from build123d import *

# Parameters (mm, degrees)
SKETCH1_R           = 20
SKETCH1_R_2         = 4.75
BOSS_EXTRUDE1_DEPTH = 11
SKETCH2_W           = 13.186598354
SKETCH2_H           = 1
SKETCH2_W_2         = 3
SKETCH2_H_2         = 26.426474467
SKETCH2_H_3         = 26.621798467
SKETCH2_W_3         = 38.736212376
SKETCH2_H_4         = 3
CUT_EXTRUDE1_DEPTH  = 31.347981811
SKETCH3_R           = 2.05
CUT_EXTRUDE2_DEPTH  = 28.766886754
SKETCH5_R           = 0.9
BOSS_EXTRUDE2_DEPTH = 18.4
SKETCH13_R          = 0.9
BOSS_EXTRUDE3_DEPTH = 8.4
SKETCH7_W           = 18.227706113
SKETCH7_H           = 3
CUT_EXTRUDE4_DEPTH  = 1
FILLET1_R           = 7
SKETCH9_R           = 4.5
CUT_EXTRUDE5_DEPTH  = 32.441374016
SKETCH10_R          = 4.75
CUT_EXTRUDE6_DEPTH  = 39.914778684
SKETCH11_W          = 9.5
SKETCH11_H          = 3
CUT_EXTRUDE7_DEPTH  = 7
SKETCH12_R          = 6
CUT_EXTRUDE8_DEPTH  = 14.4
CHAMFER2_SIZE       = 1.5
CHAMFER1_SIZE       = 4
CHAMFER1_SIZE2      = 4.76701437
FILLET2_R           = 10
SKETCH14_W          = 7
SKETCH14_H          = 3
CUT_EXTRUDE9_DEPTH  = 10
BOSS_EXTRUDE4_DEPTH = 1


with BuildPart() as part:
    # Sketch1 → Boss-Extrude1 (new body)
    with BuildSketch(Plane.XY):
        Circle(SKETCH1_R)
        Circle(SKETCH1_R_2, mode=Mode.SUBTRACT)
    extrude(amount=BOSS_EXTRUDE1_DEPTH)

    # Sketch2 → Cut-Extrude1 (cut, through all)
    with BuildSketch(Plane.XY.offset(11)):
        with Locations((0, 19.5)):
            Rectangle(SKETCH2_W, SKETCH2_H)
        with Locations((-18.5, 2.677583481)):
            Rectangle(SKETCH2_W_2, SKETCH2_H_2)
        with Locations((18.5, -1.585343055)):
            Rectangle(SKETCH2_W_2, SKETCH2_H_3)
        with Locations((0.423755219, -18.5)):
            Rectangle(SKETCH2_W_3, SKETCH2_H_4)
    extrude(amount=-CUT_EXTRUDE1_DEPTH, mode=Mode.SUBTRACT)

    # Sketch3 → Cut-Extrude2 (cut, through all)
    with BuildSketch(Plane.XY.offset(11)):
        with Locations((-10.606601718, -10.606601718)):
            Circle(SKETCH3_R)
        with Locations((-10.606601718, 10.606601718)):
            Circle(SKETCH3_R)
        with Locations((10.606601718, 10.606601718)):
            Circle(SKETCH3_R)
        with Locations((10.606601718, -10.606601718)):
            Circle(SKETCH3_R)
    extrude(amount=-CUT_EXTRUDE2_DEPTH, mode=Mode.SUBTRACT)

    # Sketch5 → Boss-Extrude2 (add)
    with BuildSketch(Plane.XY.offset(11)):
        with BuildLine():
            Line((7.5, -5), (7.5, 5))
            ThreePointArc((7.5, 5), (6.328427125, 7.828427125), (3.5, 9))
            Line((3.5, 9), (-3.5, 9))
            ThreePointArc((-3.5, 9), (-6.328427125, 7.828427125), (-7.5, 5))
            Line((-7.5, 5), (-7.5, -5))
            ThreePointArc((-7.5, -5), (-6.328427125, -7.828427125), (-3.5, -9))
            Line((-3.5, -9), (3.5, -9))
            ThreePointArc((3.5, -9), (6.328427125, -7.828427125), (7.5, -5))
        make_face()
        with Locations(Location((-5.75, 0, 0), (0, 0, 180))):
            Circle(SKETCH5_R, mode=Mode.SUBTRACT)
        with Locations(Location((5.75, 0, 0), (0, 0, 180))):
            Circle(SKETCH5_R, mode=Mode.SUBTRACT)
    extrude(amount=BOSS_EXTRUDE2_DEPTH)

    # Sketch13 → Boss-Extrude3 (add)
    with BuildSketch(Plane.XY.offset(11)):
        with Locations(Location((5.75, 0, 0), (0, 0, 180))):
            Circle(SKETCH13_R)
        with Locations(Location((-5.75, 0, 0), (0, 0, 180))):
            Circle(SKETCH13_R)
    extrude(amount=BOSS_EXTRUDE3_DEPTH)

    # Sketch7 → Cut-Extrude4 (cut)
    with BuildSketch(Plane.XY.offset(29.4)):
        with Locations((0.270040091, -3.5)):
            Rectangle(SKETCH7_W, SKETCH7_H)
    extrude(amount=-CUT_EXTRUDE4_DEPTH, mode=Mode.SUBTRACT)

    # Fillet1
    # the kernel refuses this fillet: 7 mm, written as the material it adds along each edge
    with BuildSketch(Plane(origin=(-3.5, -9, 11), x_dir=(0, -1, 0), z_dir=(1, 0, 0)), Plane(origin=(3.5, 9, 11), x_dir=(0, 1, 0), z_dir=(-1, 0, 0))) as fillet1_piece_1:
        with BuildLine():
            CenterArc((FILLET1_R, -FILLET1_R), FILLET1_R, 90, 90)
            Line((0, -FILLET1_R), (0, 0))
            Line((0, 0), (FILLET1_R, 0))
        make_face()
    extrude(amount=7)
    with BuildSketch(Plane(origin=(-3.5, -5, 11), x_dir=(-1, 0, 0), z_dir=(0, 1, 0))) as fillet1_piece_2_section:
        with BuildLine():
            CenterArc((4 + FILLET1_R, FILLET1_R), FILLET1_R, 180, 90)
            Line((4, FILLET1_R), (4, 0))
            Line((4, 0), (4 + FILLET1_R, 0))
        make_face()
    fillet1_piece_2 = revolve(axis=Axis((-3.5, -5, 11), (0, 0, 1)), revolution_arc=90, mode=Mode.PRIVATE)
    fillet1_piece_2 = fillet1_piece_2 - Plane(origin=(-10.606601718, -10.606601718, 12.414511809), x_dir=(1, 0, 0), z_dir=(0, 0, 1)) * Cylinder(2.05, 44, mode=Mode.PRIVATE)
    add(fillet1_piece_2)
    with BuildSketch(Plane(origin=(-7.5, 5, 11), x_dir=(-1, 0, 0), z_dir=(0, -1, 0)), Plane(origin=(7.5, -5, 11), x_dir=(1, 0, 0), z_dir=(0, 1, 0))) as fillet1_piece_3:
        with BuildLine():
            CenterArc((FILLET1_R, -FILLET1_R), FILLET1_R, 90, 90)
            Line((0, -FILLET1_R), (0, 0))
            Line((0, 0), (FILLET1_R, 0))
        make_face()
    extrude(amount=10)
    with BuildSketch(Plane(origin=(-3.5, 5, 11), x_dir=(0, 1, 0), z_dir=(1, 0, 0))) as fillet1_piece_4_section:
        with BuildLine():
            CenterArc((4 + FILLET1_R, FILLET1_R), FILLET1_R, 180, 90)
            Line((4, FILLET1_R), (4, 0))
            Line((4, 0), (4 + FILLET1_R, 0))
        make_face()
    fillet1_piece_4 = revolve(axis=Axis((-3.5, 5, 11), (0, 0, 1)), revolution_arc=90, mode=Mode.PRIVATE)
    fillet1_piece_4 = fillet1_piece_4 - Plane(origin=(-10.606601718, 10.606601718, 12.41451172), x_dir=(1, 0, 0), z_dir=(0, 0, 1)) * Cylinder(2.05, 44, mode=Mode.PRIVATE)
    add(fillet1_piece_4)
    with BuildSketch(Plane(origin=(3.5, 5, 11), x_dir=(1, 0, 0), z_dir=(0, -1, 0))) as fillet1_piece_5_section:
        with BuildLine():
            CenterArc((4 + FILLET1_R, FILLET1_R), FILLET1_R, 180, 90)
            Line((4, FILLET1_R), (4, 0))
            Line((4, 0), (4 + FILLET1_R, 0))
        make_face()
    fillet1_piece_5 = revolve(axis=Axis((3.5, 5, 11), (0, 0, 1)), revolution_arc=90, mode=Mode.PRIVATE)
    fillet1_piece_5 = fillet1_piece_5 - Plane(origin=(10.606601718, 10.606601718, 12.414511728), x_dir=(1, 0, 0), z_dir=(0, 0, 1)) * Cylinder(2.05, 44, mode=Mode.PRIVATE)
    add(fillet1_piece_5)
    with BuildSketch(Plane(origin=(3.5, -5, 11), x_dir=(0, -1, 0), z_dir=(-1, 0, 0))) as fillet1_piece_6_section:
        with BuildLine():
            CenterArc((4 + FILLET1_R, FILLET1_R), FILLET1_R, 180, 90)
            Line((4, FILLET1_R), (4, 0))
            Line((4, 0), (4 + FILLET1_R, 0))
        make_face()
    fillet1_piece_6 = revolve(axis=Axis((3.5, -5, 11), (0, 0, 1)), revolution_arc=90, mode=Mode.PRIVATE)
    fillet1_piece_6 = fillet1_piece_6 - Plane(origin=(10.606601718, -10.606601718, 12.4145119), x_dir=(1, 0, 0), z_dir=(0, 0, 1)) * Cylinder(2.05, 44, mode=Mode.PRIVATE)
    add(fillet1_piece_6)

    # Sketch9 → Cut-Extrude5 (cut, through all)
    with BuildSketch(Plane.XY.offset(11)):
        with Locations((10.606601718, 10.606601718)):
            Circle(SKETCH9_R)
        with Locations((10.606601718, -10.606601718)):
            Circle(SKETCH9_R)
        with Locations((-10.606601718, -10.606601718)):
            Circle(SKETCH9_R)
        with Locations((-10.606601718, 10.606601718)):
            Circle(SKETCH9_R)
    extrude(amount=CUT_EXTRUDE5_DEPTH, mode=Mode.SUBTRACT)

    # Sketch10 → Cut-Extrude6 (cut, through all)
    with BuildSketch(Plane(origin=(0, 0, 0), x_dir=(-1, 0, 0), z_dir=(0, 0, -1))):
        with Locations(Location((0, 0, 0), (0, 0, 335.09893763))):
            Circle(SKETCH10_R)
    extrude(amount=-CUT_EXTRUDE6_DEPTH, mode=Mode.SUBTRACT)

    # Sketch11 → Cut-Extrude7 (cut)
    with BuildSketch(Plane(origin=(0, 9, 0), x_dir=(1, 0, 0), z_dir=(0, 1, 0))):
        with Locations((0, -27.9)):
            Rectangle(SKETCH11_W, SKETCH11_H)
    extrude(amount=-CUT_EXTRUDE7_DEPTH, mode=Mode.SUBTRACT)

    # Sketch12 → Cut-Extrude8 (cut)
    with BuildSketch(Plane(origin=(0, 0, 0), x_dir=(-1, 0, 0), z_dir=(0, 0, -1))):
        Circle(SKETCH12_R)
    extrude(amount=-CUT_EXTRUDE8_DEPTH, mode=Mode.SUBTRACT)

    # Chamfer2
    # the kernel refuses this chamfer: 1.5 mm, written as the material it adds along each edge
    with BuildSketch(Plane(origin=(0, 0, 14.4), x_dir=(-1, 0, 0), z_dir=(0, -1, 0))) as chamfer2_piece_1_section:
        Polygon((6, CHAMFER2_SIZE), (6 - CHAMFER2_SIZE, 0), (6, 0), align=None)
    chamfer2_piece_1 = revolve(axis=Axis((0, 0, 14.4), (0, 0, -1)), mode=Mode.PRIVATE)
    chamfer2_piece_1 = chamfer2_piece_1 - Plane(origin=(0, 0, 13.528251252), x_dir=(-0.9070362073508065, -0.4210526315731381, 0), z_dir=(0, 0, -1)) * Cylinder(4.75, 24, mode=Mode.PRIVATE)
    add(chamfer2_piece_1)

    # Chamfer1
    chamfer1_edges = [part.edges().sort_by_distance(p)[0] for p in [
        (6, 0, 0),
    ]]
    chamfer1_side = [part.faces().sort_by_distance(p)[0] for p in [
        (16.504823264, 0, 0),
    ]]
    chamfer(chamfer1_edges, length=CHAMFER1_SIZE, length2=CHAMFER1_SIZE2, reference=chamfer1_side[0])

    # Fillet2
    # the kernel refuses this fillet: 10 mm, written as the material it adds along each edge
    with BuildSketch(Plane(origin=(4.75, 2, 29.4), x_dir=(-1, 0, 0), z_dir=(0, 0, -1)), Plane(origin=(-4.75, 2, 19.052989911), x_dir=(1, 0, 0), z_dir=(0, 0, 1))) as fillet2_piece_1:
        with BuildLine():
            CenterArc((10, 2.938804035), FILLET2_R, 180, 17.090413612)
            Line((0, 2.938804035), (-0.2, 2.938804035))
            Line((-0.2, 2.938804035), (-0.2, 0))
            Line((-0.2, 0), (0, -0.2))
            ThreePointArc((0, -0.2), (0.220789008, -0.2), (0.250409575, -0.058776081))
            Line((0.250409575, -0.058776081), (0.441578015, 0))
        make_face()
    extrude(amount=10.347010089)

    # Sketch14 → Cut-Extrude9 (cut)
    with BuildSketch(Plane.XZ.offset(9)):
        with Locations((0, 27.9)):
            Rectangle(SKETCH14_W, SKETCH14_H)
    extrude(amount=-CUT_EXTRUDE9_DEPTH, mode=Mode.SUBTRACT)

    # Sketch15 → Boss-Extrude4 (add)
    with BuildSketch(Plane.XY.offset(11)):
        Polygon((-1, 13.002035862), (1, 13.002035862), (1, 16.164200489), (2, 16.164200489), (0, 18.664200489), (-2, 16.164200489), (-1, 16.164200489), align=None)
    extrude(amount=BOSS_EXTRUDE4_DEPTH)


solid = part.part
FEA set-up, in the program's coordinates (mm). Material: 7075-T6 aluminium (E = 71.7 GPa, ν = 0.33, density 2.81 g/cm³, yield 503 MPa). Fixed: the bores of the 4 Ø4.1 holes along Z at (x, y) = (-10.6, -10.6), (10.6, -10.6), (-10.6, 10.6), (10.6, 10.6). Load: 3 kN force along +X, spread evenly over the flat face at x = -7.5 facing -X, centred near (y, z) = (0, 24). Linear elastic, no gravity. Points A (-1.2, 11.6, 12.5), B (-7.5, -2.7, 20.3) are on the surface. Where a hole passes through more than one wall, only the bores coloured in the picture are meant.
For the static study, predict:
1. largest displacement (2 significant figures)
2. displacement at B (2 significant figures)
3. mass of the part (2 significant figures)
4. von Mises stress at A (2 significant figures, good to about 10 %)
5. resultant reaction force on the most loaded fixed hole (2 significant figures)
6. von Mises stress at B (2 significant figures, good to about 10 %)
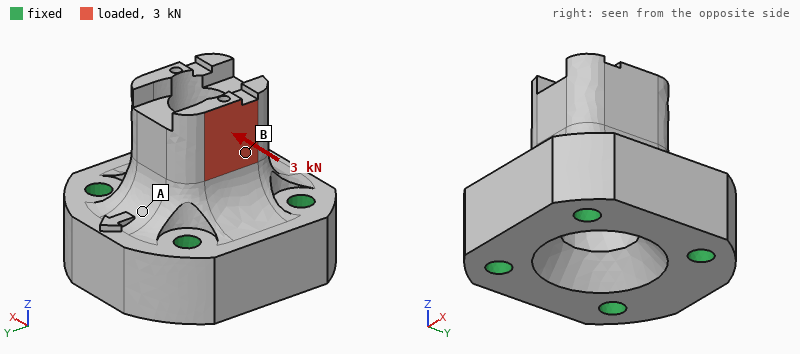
57 µm
21 µm
38 g
18 MPa
1.4 kN
54 MPa
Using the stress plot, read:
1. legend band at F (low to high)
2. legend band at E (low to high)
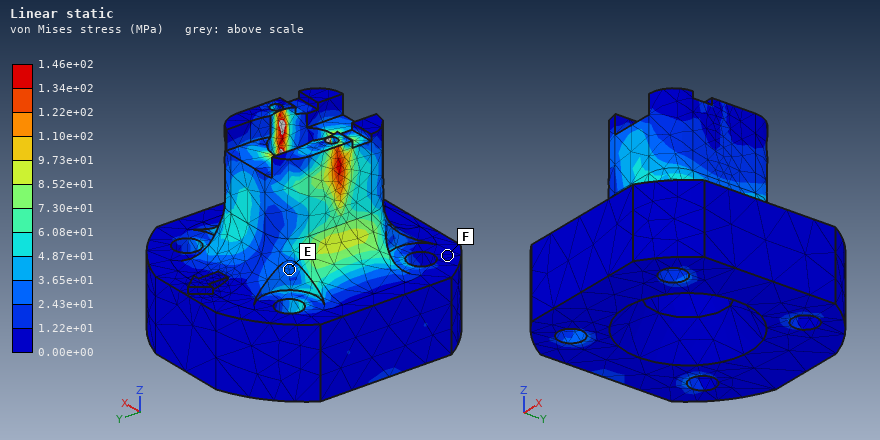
0.00e+00 to 1.22e+01 MPa
2.43e+01 to 3.65e+01 MPa
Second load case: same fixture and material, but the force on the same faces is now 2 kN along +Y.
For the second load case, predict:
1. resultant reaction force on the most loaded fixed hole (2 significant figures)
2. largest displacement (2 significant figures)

1.0 kN
25 µm
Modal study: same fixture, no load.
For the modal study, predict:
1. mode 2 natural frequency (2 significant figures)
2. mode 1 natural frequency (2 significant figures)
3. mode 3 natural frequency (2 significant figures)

28 kHz
27 kHz
42 kHz
